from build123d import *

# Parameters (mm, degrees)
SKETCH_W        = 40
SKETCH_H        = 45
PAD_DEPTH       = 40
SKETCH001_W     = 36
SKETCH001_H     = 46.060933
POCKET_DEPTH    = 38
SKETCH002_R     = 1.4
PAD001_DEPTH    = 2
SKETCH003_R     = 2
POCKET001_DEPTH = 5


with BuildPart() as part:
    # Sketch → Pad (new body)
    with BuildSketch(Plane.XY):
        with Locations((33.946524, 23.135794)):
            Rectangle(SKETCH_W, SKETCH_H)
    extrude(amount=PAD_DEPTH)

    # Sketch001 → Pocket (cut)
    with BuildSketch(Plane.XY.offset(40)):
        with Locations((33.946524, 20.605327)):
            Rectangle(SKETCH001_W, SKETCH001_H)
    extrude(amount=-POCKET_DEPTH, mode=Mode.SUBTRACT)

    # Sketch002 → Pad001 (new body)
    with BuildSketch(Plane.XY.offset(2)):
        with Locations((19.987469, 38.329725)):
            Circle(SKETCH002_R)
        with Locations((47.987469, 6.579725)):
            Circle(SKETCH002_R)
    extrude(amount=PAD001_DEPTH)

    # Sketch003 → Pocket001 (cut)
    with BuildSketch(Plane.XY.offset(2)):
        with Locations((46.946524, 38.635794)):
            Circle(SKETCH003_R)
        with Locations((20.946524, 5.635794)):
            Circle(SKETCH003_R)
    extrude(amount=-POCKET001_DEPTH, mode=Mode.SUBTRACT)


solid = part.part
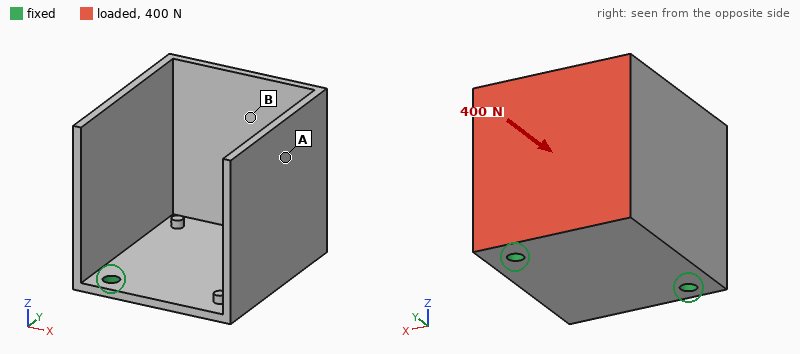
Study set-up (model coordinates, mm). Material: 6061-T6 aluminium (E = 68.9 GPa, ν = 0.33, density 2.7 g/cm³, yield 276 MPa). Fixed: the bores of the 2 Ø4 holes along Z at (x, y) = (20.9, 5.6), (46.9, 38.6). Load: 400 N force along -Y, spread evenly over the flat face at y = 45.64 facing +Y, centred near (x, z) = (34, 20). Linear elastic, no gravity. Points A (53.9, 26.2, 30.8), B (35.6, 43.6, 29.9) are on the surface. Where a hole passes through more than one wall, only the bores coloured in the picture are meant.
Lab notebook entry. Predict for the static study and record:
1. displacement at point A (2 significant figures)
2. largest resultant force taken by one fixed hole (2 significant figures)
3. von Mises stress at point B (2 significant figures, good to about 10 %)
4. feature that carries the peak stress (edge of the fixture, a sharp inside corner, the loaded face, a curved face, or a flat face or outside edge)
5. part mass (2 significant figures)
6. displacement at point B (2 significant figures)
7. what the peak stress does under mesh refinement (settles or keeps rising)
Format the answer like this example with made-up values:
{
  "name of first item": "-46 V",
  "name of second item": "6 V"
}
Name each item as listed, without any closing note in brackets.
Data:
{
  "displacement at point A": "0.23 mm",
  "largest resultant force taken by one fixed hole": "230 N",
  "von Mises stress at point B": "32 MPa",
  "feature that carries the peak stress": "edge of the fixture",
  "part mass": "36 g",
  "displacement at point B": "0.23 mm",
  "what the peak stress does under mesh refinement": "keeps rising"
}
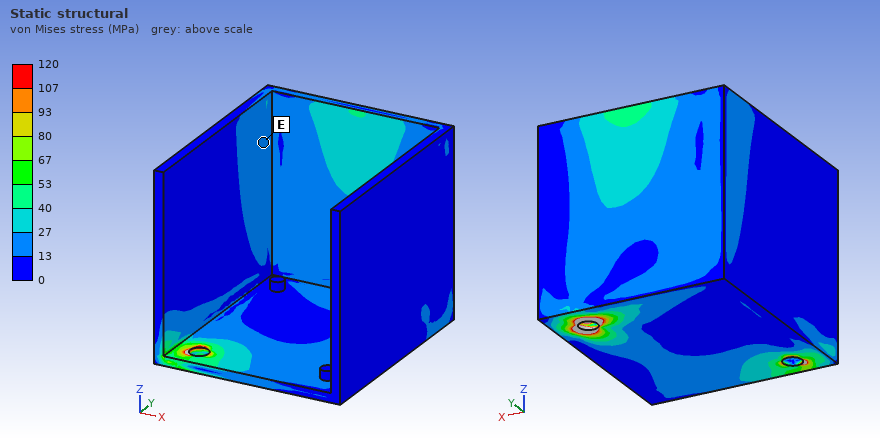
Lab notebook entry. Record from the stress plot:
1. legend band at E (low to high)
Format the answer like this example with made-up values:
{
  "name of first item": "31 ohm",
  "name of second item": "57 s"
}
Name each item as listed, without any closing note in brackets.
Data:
{
  "legend band at E": "13 to 27 MPa"
}
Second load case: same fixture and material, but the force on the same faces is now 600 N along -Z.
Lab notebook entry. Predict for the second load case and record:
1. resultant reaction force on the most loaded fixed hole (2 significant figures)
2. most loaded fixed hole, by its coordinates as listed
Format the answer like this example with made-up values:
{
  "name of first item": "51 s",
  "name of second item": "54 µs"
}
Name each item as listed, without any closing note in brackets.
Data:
{
  "resultant reaction force on the most loaded fixed hole": "530 N",
  "most loaded fixed hole, by its coordinates as listed": "(46.9, 38.6)"
}
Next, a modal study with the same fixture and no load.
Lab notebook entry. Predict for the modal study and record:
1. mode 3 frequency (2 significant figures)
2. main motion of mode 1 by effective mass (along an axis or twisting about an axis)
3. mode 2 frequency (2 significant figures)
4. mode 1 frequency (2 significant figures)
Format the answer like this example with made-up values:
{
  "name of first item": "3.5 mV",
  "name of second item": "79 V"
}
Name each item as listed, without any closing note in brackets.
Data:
{
  "mode 3 frequency": "1600 Hz",
  "main motion of mode 1 by effective mass": "along X",
  "mode 2 frequency": "1300 Hz",
  "mode 1 frequency": "940 Hz"
}
